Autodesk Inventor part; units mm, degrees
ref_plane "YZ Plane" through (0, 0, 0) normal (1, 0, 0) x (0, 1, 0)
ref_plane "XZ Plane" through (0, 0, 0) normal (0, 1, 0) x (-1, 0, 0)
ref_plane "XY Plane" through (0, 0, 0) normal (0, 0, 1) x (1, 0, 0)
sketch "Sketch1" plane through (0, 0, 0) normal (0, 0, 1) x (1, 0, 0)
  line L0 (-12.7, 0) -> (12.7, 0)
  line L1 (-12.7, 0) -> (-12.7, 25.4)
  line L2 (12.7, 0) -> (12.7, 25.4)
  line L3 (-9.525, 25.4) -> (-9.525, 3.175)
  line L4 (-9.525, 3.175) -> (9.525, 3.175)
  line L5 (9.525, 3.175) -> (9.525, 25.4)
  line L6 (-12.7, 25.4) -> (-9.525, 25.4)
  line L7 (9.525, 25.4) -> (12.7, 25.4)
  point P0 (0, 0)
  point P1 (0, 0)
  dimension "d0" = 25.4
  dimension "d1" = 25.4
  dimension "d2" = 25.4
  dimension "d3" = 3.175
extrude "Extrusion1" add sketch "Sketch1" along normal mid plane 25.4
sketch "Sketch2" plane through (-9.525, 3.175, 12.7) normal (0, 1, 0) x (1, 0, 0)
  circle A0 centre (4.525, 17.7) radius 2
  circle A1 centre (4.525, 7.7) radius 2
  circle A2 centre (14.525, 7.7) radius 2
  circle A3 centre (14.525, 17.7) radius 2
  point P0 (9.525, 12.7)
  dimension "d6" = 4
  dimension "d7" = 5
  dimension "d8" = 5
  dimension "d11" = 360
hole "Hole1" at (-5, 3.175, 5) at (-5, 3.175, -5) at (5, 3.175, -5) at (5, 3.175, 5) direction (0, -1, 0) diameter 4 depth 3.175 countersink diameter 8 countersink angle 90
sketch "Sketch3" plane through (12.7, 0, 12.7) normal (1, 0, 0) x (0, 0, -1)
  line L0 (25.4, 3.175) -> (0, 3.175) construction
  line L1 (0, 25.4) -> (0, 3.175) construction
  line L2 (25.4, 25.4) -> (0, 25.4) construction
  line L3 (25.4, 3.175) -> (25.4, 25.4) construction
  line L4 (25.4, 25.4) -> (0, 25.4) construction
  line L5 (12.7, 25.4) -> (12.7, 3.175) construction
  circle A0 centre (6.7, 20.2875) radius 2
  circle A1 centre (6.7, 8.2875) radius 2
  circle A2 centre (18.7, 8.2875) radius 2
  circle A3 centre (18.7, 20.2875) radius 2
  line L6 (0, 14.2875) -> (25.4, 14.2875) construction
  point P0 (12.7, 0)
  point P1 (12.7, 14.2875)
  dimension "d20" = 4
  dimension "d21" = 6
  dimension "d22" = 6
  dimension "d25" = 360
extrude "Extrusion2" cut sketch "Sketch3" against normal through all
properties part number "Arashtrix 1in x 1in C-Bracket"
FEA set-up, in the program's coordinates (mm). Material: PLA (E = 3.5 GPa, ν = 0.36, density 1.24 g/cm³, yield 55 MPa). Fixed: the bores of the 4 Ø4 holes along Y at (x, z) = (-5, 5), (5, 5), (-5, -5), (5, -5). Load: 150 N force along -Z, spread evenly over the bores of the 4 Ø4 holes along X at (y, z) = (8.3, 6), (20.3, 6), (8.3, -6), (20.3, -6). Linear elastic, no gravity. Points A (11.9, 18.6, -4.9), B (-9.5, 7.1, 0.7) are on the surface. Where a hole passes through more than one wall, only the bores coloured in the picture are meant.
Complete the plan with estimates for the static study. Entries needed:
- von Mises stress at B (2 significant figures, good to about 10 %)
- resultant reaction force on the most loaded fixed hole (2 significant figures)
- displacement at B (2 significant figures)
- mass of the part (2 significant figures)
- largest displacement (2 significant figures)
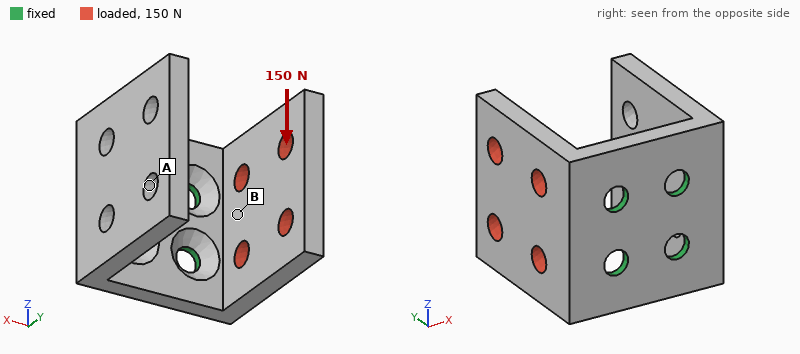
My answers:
11 MPa
210 N
0.11 mm
6.2 g
0.48 mm
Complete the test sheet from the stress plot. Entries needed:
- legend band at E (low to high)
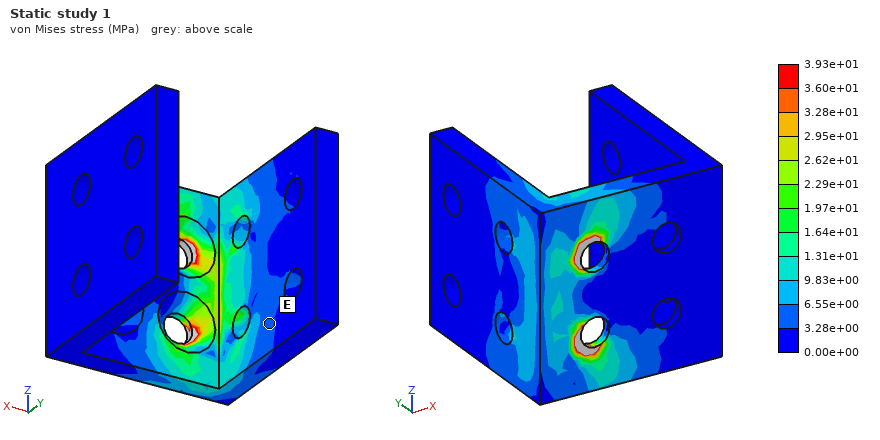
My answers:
3.28e+00 to 6.55e+00 MPa
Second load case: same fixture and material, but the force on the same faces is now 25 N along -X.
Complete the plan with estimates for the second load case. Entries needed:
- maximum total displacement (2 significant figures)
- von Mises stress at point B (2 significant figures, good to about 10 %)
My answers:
0.47 mm
5.0 MPa
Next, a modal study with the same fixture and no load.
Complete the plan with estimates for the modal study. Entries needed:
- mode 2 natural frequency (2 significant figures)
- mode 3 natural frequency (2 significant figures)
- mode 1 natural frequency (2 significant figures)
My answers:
1000 Hz
2200 Hz
990 Hz
